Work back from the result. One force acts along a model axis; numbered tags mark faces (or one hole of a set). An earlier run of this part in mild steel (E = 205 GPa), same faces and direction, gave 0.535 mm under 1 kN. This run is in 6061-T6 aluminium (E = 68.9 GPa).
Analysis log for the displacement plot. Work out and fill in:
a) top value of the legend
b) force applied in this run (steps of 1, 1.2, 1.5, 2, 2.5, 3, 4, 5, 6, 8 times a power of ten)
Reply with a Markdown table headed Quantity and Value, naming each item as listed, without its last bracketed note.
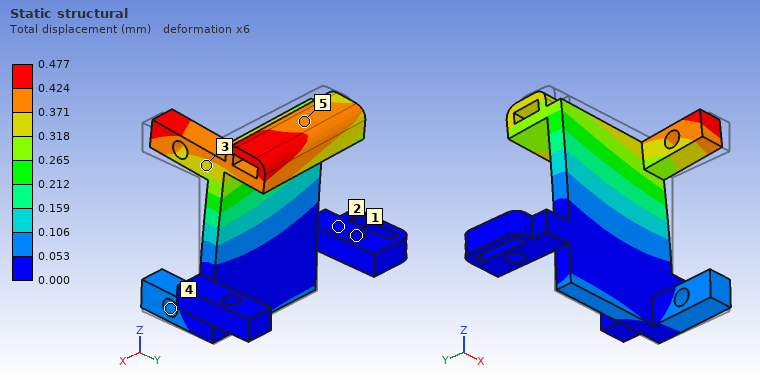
| Quantity | Value |
|---|---|
| top value of the legend | 0.477 mm |
| force applied in this run | 300 N |
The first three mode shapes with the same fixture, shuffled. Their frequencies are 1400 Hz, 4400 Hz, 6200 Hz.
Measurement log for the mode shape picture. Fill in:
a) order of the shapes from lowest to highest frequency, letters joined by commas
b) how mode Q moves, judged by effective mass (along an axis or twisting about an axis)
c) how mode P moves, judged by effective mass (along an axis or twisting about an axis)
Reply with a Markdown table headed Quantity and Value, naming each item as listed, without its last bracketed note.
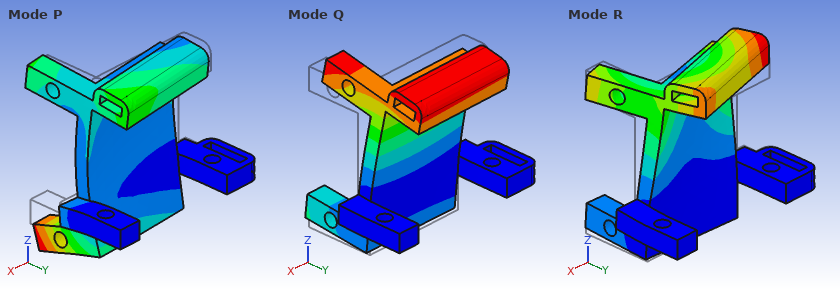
| Quantity | Value |
|---|---|
| order of the shapes from lowest to highest frequency, letters joined by commas | Q, R, P |
| how mode Q moves, judged by effective mass | along Y |
| how mode P moves, judged by effective mass | along Z |
